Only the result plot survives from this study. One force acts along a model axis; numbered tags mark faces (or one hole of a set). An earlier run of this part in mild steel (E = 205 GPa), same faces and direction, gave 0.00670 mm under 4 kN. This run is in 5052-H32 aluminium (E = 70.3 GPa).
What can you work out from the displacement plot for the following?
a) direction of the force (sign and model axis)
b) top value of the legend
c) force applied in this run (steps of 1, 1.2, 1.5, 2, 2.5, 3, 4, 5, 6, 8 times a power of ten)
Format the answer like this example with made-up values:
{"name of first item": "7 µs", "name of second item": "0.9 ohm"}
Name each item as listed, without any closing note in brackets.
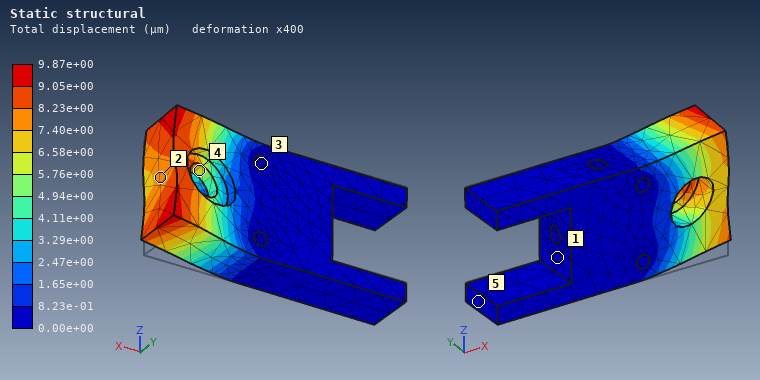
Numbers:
{"direction of the force": "+Z", "top value of the legend": "9.87e+00 µm", "force applied in this run": "2 kN"}
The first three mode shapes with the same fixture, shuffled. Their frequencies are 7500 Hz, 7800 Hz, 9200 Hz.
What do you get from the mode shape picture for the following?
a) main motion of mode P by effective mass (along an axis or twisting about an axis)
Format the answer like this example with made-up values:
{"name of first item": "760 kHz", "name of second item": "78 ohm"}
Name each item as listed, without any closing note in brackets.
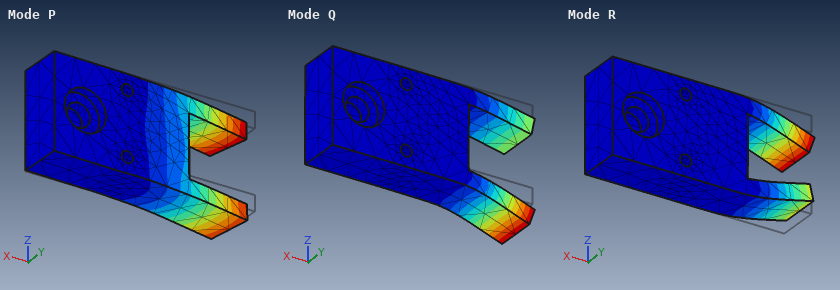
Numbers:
{"main motion of mode P by effective mass": "along Y"}
